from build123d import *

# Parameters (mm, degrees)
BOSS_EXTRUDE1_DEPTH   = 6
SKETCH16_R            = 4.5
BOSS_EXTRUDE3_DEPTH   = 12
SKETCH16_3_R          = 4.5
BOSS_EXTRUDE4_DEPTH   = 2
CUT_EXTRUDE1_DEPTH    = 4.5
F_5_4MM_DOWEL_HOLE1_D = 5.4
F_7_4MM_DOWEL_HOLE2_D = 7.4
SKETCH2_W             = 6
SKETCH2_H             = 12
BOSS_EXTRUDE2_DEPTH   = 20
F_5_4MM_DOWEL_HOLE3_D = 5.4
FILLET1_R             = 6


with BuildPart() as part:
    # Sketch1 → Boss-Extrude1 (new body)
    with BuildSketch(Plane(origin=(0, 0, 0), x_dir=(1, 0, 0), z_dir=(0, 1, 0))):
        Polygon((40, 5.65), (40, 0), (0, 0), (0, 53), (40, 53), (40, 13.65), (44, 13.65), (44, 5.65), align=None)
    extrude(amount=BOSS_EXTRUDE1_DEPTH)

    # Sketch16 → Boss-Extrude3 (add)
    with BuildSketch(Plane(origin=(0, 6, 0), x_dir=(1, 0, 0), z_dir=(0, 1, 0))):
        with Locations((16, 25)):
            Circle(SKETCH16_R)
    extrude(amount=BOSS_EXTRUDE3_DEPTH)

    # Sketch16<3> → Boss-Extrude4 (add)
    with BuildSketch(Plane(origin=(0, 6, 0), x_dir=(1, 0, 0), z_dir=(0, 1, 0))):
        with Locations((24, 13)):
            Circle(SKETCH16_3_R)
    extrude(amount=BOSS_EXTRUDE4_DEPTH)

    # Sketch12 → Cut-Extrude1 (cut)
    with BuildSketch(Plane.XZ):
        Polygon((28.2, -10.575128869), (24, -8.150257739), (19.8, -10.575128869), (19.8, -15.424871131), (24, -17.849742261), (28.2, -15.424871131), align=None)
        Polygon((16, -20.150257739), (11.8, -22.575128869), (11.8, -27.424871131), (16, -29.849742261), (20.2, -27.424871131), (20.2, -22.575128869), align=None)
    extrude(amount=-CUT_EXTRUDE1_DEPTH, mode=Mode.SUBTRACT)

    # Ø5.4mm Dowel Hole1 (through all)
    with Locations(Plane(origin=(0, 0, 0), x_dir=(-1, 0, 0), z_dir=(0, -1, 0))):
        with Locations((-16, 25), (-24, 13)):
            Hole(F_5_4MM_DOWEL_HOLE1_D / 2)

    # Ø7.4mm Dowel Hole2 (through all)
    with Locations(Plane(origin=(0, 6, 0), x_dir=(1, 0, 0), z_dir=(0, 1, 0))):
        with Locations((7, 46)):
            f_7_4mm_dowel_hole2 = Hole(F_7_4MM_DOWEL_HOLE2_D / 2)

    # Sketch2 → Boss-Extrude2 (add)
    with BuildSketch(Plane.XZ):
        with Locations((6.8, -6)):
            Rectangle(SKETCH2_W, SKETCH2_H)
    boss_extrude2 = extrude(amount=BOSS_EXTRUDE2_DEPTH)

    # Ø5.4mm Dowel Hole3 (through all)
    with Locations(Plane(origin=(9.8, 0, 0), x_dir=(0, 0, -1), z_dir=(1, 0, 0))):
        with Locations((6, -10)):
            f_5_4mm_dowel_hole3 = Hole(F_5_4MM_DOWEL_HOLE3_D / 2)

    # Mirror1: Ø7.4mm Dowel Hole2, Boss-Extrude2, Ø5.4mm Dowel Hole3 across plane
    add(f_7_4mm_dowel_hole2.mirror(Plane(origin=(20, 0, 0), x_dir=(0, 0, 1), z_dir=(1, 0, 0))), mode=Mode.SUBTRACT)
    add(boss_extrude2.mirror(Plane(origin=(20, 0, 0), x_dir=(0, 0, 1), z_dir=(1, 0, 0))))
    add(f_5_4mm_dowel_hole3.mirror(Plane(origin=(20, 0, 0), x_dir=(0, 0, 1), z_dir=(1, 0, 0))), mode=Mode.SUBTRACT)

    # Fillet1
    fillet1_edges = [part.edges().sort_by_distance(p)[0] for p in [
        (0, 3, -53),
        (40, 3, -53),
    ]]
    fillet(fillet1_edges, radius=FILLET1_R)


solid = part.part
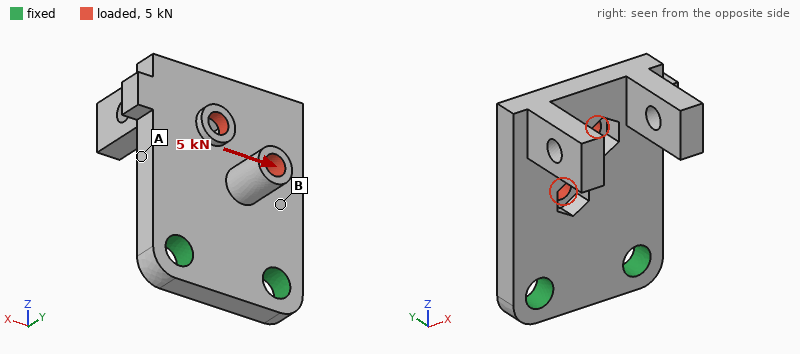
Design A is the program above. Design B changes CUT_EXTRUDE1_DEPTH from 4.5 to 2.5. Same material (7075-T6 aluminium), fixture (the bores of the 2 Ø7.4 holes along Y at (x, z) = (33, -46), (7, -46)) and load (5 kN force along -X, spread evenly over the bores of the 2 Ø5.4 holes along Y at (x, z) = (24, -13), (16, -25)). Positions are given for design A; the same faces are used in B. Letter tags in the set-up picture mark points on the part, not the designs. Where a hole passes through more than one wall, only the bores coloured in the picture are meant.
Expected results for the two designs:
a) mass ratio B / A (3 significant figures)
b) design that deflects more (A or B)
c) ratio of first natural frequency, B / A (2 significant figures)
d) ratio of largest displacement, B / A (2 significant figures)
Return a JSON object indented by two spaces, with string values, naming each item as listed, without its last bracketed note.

{
  "mass ratio B / A": "1.01",
  "design that deflects more": "A",
  "ratio of first natural frequency, B / A": "1.0",
  "ratio of largest displacement, B / A": "0.77"
}
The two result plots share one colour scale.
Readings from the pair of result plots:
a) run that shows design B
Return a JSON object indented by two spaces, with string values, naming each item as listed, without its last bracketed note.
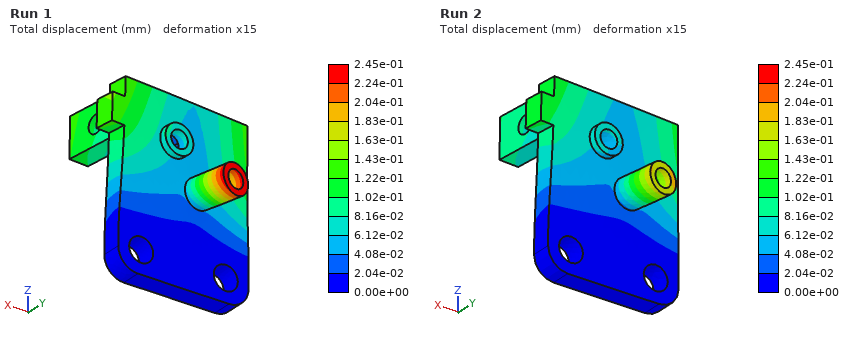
{
  "run that shows design B": "Run 2"
}
